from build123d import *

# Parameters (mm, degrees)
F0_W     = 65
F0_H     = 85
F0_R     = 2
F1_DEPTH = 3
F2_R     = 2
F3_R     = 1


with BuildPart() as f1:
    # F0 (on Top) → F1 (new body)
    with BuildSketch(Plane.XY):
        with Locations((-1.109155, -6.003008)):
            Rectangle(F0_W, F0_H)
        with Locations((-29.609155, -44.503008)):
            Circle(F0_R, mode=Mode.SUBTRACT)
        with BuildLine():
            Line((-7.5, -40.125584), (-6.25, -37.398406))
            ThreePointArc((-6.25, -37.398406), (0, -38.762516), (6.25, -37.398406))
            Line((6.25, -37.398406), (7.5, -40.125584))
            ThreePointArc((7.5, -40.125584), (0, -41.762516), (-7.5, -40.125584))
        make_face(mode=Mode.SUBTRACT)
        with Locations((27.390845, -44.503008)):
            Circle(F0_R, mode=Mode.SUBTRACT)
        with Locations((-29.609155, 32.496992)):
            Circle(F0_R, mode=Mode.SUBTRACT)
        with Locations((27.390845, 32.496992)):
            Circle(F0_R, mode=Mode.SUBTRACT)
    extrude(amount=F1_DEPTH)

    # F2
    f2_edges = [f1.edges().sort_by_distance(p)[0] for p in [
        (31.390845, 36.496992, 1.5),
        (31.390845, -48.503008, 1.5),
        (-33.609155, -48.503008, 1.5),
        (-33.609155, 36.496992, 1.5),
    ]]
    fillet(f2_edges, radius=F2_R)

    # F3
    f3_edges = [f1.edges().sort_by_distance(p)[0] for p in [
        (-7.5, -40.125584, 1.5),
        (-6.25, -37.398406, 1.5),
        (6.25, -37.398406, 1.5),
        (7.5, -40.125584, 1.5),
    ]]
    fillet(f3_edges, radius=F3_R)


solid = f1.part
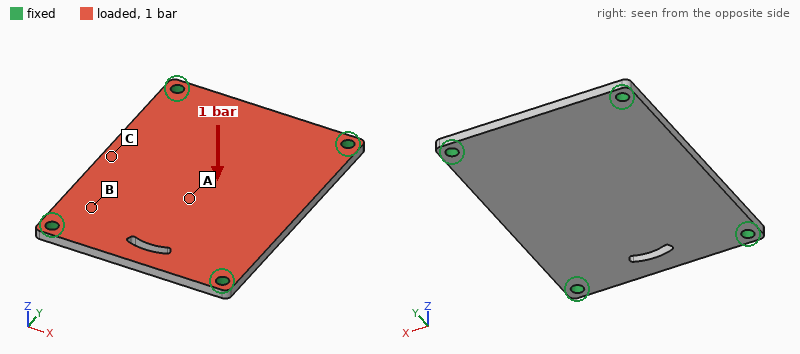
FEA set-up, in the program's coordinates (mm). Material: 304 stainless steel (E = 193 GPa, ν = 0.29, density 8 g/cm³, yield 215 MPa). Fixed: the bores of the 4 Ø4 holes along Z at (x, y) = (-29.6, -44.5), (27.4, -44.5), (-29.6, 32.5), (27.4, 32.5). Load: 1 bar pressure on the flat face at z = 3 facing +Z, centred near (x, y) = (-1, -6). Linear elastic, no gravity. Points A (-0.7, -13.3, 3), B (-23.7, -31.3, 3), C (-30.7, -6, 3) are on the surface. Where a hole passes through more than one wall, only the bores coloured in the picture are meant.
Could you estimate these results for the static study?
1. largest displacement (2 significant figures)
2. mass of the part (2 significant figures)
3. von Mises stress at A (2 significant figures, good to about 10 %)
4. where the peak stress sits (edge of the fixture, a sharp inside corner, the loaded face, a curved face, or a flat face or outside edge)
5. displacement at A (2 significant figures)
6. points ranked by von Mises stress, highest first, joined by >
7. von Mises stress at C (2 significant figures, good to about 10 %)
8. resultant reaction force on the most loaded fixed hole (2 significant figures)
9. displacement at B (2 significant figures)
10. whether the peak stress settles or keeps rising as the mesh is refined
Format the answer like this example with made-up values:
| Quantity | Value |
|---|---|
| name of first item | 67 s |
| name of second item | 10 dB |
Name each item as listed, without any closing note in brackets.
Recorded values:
| Quantity | Value |
|---|---|
| largest displacement | 37 µm |
| mass of the part | 130 g |
| von Mises stress at A | 17 MPa |
| where the peak stress sits | edge of the fixture |
| displacement at A | 36 µm |
| points ranked by von Mises stress, highest first, joined by > | C > A > B |
| von Mises stress at C | 23 MPa |
| resultant reaction force on the most loaded fixed hole | 140 N |
| displacement at B | 14 µm |
| whether the peak stress settles or keeps rising as the mesh is refined | keeps rising |
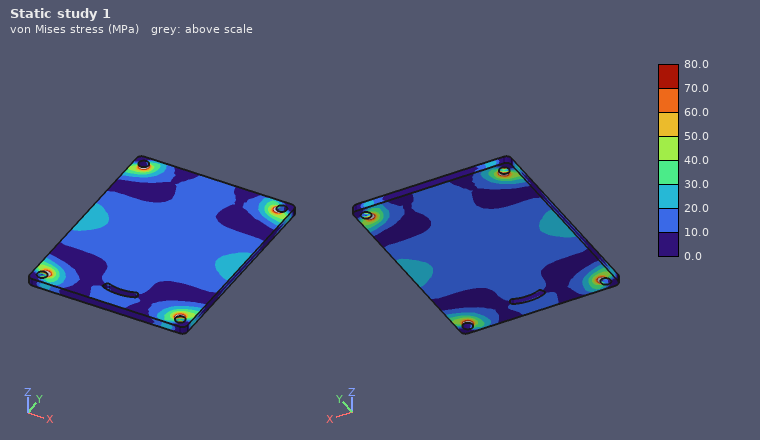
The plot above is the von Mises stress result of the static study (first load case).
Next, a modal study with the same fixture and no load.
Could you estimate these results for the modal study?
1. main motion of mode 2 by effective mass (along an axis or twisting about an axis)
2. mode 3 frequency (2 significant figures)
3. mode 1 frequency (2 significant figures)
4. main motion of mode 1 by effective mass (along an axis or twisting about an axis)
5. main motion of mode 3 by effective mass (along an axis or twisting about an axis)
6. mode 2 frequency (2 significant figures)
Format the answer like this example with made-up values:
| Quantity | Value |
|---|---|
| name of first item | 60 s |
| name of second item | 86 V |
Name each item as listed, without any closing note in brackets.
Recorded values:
| Quantity | Value |
|---|---|
| main motion of mode 2 by effective mass | twisting about Y |
| mode 3 frequency | 4400 Hz |
| mode 1 frequency | 2000 Hz |
| main motion of mode 1 by effective mass | along Z |
| main motion of mode 3 by effective mass | twisting about X |
| mode 2 frequency | 3200 Hz |
